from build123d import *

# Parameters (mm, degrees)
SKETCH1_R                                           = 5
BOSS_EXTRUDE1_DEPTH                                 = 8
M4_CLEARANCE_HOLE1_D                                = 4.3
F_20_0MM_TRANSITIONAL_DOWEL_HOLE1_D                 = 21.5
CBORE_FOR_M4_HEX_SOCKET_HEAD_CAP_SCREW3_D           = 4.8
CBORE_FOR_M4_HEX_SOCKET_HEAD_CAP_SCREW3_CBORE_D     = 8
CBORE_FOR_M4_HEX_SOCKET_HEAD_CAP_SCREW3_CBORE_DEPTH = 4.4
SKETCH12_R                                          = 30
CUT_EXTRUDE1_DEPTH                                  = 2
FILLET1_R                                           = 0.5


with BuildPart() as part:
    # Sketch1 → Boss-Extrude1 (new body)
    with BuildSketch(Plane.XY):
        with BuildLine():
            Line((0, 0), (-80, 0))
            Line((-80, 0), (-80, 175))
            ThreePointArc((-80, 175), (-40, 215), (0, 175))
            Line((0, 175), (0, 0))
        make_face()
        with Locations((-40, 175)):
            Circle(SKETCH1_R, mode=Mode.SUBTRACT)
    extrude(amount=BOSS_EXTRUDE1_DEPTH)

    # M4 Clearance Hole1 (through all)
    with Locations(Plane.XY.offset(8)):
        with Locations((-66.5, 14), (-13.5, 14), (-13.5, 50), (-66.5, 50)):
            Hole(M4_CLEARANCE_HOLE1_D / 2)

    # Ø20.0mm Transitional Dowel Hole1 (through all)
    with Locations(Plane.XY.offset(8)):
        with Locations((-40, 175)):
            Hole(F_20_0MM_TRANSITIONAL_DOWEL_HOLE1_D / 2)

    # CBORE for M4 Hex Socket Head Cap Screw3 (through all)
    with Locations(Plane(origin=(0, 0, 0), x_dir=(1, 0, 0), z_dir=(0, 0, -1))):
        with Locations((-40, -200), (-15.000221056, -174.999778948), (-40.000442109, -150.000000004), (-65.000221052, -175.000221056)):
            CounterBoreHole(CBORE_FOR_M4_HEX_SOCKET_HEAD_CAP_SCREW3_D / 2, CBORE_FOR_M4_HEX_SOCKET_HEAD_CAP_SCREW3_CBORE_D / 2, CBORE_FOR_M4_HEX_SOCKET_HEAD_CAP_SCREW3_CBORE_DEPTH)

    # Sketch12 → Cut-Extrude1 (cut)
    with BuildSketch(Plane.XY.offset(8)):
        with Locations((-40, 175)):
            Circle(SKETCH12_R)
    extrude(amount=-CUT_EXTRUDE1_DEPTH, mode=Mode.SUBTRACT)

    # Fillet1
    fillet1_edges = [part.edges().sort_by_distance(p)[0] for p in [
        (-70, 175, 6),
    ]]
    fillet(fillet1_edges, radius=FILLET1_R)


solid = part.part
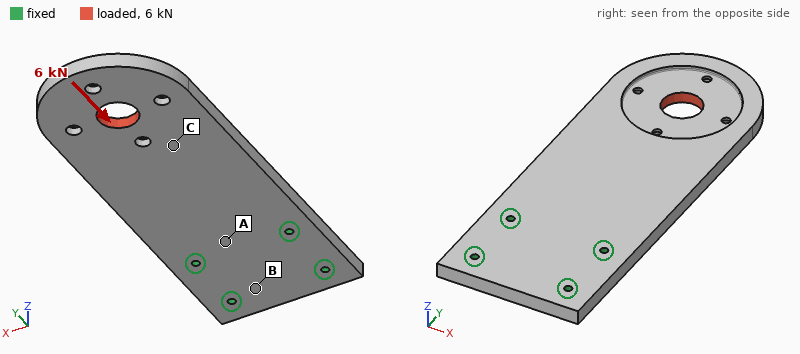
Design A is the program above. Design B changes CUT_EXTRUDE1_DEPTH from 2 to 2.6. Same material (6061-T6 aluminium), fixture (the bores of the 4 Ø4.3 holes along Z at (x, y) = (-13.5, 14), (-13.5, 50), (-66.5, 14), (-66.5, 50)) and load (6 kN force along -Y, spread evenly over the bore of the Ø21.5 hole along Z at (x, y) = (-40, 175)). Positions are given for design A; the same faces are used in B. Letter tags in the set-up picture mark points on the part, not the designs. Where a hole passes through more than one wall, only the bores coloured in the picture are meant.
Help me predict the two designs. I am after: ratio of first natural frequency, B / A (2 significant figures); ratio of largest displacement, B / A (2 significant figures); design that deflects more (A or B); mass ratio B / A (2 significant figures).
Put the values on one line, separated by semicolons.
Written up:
1.0; 1.3; B; 0.99
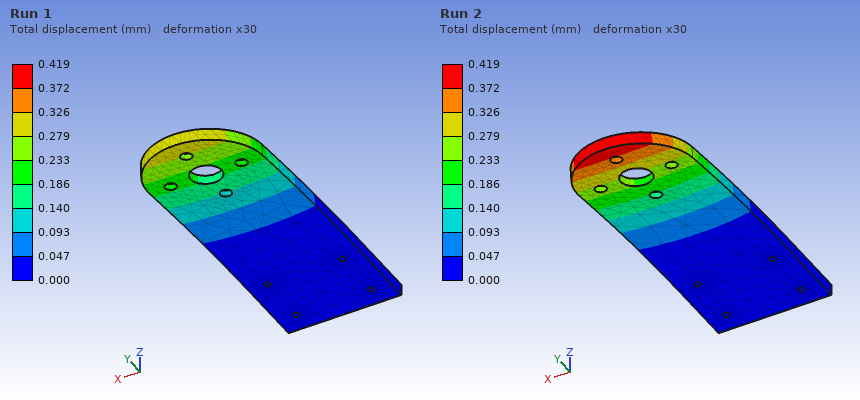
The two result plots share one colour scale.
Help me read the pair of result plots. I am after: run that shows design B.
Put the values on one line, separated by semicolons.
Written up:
Run 2
